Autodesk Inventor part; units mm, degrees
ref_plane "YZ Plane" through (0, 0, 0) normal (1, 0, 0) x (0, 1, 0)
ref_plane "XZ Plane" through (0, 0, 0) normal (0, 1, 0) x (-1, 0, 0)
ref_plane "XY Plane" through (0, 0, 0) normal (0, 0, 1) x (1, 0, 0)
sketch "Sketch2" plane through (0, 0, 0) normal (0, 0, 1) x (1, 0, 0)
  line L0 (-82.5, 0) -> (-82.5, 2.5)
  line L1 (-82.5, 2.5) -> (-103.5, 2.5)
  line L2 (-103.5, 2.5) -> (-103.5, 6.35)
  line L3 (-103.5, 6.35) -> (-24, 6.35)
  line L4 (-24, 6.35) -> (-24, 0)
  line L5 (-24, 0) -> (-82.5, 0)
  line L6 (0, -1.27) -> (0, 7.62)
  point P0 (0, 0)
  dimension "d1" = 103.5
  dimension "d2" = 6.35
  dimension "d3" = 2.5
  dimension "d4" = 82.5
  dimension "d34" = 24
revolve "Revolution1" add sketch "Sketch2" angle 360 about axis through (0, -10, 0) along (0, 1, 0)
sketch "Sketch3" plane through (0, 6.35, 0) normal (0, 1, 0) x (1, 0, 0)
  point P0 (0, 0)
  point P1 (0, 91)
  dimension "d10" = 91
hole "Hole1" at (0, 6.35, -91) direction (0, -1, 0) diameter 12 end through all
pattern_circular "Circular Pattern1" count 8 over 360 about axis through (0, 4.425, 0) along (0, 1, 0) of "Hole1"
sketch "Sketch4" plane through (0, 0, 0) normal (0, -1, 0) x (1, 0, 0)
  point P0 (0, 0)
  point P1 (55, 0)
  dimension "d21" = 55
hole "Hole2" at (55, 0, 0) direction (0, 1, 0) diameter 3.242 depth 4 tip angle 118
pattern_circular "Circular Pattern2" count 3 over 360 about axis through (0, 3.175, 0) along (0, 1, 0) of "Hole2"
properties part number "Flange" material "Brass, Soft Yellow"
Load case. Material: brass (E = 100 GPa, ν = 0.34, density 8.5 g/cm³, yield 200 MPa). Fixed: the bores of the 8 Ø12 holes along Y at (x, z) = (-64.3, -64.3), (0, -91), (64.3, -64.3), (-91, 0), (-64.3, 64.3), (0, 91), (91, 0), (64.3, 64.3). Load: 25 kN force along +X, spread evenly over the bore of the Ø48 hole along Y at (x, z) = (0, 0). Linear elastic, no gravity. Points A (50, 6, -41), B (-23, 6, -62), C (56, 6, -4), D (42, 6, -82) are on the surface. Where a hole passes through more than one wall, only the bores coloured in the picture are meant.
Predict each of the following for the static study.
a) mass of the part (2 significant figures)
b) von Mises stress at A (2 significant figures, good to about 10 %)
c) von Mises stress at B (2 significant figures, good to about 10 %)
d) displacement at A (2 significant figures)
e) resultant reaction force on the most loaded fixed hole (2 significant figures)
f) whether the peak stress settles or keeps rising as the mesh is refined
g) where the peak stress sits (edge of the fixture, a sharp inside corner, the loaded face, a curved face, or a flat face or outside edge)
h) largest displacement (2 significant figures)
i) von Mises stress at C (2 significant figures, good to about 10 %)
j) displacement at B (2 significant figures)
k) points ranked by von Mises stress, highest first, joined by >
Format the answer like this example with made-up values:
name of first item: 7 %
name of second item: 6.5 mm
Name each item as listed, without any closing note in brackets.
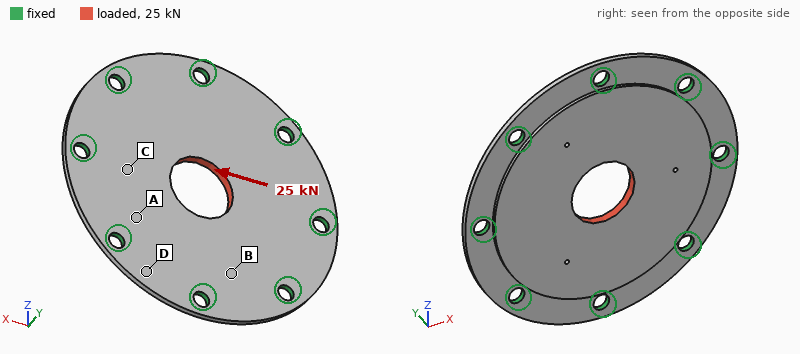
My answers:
mass of the part: 1.4 kg
von Mises stress at A: 20 MPa
von Mises stress at B: 10 MPa
displacement at A: 11 µm
resultant reaction force on the most loaded fixed hole: 5.0 kN
whether the peak stress settles or keeps rising as the mesh is refined: keeps rising
where the peak stress sits: edge of the fixture
largest displacement: 21 µm
von Mises stress at C: 26 MPa
displacement at B: 6.2 µm
points ranked by von Mises stress, highest first, joined by >: C > A > B > D
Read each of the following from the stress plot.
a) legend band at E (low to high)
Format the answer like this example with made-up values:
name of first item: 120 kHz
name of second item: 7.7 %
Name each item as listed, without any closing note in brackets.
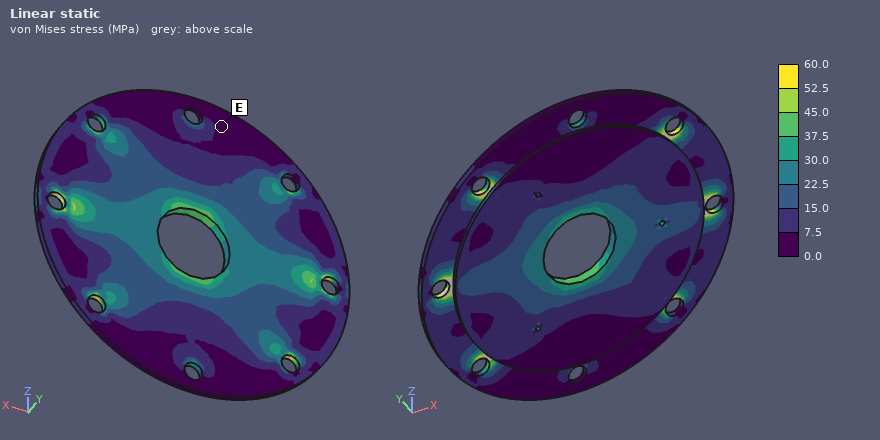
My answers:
legend band at E: 0.0 to 7.5 MPa
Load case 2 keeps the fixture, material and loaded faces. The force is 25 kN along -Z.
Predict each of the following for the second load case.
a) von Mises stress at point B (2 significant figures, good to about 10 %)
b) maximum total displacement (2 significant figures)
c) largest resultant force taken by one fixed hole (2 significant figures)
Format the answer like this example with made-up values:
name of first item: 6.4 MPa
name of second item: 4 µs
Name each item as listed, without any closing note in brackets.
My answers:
von Mises stress at point B: 15 MPa
maximum total displacement: 21 µm
largest resultant force taken by one fixed hole: 5.0 kN
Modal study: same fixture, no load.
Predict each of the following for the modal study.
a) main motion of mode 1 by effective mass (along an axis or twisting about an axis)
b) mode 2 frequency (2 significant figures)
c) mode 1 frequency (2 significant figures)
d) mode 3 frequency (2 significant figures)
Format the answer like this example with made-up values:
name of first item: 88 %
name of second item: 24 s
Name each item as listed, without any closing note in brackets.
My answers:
main motion of mode 1 by effective mass: along Y
mode 2 frequency: 2000 Hz
mode 1 frequency: 1000 Hz
mode 3 frequency: 2000 Hz
